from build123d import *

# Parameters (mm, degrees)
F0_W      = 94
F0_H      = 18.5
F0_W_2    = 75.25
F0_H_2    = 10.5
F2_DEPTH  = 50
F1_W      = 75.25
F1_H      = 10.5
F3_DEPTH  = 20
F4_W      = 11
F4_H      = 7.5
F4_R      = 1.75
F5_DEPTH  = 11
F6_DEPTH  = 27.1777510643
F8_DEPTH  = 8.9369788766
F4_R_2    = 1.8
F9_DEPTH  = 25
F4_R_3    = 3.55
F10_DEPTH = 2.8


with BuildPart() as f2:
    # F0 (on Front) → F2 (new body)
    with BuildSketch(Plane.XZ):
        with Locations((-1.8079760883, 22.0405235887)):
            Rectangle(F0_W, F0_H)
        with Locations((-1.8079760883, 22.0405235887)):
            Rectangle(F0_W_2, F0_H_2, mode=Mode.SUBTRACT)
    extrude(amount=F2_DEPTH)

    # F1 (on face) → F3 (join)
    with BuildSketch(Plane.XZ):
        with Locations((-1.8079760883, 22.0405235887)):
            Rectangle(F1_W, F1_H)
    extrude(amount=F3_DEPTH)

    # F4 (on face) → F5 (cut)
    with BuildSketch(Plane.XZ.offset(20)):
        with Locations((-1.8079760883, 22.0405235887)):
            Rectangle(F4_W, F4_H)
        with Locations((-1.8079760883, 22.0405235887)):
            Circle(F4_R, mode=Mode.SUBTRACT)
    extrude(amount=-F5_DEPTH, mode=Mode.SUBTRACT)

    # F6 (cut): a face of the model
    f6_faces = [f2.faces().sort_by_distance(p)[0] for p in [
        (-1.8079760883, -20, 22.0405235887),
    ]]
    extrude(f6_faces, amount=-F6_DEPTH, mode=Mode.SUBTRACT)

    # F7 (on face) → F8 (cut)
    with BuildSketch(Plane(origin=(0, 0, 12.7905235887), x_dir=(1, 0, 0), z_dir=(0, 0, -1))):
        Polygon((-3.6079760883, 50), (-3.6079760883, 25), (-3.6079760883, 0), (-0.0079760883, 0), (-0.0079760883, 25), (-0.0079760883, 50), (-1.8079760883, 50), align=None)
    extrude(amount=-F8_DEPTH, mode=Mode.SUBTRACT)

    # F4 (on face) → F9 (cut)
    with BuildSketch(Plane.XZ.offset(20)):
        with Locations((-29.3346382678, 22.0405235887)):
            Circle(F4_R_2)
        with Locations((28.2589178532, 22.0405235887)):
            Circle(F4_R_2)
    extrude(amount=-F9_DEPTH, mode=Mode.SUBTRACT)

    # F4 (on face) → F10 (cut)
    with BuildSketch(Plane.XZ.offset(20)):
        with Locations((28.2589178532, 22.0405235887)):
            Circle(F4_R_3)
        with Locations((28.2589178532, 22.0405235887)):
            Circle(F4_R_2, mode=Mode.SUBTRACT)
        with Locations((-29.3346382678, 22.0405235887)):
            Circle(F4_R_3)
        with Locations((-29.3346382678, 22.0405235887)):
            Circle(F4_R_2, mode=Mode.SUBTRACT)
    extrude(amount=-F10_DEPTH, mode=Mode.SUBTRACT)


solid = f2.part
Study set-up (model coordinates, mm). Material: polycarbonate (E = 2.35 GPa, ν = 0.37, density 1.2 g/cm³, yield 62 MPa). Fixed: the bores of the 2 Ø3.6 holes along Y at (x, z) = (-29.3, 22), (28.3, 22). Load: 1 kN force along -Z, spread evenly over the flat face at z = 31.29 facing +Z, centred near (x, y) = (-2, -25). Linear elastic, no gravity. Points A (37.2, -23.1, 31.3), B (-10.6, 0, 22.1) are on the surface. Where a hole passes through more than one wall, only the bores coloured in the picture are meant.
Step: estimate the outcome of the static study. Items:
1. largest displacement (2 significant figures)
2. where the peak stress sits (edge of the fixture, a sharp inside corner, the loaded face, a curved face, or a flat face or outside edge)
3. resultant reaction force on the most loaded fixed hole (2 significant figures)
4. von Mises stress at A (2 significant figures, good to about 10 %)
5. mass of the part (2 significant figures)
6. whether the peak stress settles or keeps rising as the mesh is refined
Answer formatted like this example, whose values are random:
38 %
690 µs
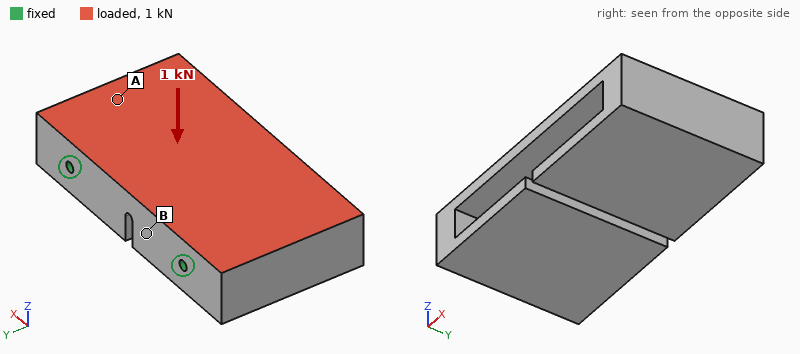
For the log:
1.2 mm
edge of the fixture
560 N
3.9 MPa
73 g
keeps rising
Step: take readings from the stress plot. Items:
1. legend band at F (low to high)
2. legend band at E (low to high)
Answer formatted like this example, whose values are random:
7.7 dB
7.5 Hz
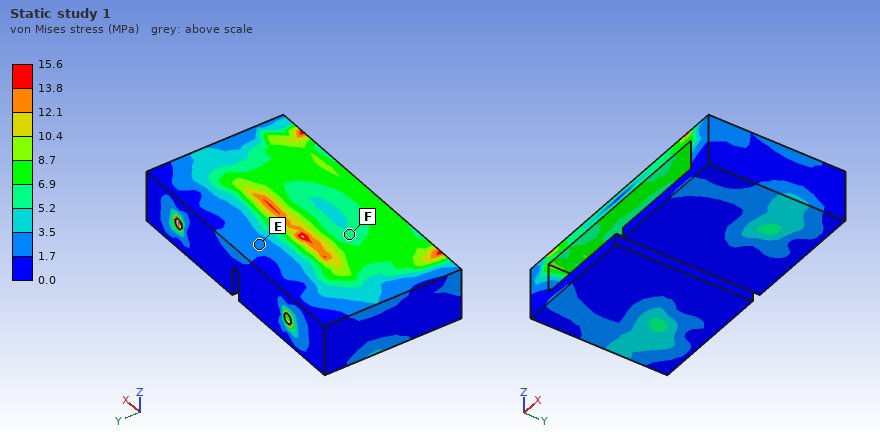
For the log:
5.2 to 6.9 MPa
1.7 to 3.5 MPa
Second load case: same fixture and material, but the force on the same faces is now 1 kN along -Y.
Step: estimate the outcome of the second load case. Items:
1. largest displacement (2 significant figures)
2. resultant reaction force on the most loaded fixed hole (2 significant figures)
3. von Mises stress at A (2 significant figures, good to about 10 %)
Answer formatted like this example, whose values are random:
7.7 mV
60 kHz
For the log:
0.31 mm
520 N
1.9 MPa
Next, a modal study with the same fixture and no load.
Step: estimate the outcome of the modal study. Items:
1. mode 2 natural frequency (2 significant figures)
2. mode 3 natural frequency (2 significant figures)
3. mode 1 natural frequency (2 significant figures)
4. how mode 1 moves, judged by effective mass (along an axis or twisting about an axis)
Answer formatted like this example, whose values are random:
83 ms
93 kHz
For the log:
1300 Hz
1500 Hz
1200 Hz
along Z
